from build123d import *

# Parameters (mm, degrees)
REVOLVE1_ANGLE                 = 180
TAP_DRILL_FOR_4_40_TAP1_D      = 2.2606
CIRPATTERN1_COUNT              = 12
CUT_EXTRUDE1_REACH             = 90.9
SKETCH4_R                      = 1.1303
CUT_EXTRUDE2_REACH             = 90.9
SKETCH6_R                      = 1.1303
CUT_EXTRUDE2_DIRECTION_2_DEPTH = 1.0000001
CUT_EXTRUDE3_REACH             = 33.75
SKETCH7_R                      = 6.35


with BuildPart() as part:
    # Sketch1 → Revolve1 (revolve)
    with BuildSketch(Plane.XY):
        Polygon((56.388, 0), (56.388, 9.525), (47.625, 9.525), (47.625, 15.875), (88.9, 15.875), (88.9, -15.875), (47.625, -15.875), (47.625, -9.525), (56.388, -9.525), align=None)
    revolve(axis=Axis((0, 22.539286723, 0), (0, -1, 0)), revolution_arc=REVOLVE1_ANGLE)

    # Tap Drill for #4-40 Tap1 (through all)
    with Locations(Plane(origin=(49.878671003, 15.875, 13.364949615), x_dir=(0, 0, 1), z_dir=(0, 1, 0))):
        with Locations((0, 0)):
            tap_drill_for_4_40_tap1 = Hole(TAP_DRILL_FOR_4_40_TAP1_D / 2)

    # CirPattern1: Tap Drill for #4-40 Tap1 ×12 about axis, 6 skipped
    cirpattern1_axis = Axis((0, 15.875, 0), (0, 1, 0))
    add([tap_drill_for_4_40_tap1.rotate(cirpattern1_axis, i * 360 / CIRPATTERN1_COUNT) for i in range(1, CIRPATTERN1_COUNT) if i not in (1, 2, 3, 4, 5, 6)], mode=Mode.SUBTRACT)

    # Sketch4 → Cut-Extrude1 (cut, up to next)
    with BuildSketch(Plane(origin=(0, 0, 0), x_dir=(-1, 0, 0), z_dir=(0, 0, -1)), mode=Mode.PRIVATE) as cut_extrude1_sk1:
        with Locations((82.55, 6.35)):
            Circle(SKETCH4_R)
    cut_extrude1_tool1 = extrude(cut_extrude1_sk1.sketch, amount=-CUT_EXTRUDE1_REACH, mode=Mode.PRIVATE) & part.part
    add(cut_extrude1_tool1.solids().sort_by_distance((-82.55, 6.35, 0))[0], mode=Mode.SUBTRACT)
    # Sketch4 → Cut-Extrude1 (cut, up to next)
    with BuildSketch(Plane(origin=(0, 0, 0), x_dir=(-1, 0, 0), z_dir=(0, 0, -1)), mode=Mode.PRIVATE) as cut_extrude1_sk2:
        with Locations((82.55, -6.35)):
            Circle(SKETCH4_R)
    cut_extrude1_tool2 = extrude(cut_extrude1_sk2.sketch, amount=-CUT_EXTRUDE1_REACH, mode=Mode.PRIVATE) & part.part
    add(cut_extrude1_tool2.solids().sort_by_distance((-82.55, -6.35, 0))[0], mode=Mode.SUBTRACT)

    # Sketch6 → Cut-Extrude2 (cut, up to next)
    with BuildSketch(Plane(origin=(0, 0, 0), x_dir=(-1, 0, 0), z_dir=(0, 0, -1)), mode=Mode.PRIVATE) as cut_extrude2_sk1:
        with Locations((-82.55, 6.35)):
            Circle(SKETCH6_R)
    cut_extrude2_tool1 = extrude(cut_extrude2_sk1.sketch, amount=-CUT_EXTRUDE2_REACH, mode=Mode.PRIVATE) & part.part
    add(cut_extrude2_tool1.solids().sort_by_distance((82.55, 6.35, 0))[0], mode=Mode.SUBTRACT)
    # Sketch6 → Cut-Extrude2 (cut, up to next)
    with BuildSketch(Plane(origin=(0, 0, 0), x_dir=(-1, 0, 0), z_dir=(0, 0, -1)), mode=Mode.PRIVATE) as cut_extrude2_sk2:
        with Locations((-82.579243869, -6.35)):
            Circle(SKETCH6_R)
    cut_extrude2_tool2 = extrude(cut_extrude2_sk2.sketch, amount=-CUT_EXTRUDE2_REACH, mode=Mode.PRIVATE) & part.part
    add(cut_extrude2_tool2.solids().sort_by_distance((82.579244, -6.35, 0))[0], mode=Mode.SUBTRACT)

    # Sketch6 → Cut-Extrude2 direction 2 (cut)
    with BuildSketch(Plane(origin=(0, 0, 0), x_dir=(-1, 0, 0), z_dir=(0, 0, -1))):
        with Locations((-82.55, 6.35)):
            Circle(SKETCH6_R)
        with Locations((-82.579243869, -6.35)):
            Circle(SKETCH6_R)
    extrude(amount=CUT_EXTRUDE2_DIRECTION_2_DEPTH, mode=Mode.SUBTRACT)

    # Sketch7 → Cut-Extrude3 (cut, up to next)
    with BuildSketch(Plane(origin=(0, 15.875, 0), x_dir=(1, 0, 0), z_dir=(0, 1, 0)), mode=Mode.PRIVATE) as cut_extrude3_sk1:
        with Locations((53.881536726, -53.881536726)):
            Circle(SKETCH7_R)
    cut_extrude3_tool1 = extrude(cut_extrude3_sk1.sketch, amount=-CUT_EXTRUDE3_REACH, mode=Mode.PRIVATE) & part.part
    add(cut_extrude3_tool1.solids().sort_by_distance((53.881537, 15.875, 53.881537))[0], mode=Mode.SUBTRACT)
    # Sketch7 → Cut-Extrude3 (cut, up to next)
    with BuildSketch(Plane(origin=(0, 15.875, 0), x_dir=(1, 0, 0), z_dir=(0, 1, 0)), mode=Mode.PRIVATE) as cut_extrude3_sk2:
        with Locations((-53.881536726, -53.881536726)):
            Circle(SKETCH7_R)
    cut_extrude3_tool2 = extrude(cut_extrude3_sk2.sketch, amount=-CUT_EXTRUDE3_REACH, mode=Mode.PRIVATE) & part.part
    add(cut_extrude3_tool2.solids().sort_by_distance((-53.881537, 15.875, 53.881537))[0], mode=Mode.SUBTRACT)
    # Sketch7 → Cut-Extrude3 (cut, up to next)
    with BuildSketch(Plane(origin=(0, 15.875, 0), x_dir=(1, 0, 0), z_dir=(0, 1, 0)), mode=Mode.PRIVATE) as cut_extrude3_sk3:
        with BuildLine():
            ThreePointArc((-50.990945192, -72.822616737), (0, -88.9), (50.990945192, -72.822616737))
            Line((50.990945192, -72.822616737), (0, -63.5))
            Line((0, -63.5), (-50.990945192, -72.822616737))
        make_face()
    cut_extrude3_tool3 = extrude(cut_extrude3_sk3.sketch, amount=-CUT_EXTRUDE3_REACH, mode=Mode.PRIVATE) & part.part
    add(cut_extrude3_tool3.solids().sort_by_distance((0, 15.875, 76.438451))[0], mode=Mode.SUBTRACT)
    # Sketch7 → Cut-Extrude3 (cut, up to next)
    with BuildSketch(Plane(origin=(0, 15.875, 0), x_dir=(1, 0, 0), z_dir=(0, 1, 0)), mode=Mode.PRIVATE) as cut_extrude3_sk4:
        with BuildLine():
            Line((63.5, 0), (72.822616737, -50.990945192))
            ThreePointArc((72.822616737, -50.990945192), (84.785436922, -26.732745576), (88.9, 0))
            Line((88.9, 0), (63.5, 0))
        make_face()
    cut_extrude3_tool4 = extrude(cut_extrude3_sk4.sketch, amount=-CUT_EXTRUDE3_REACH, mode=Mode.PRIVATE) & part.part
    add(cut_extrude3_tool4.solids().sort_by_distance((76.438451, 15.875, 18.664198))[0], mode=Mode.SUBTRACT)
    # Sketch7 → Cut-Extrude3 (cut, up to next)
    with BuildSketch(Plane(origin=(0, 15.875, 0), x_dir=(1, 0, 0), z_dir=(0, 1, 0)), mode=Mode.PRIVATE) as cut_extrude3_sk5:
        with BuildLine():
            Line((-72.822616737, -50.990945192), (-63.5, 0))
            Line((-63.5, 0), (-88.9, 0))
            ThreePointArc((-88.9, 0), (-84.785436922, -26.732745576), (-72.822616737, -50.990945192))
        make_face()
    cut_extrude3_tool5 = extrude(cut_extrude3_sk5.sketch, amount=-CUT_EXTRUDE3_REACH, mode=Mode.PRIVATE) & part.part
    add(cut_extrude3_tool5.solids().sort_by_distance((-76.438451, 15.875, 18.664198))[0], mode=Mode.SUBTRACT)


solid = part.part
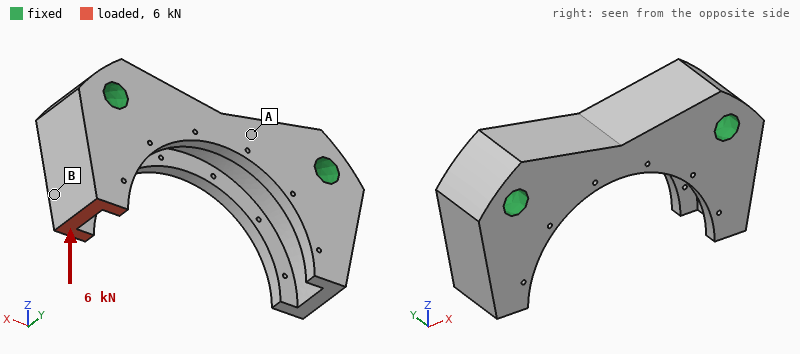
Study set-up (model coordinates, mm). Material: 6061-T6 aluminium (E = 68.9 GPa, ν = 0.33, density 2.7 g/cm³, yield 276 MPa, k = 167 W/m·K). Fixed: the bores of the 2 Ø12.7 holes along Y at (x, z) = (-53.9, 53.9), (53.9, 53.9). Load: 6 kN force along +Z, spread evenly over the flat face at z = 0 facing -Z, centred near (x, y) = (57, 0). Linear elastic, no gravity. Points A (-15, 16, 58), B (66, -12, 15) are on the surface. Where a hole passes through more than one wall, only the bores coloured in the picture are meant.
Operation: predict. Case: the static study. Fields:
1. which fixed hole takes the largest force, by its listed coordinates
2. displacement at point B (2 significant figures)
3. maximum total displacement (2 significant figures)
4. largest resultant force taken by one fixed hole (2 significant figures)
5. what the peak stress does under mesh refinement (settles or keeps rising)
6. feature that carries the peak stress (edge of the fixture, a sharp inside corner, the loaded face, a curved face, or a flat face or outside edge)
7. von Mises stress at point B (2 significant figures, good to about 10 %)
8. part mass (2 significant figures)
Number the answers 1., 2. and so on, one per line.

1. (53.9, 53.9)
2. 6.5 µm
3. 9.7 µm
4. 6.0 kN
5. keeps rising
6. a sharp inside corner
7. 10 MPa
8. 390 g
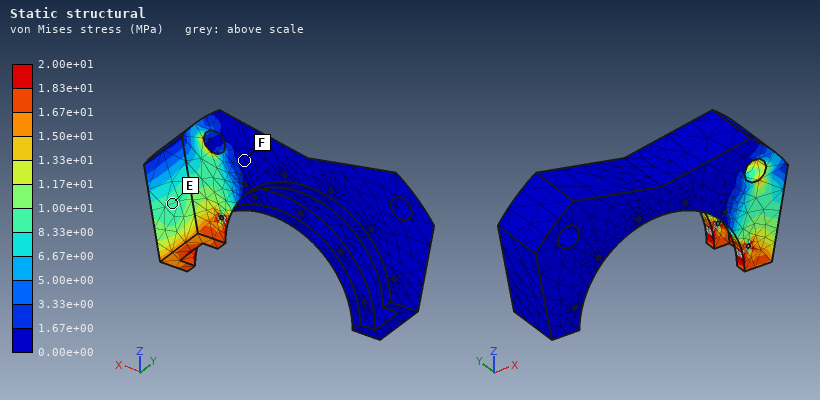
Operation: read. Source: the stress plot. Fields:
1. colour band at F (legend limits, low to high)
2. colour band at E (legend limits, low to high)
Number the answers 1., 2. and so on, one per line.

1. 0.00e+00 to 1.67e+00 MPa
2. 8.33e+00 to 1.00e+01 MPa
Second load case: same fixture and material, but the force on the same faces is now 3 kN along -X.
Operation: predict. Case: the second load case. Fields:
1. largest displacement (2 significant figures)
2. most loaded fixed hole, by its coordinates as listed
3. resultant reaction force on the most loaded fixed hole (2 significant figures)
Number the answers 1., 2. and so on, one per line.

1. 60 µm
2. (53.9, 53.9)
3. 3.1 kN
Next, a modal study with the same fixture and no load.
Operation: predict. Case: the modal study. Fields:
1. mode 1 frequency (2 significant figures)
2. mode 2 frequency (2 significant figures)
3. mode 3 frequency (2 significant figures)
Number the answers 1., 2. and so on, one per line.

1. 7900 Hz
2. 9700 Hz
3. 10000 Hz
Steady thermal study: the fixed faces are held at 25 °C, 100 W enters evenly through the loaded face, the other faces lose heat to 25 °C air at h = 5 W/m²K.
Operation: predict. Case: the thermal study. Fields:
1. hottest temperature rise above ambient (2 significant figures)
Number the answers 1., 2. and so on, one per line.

1. 52 K
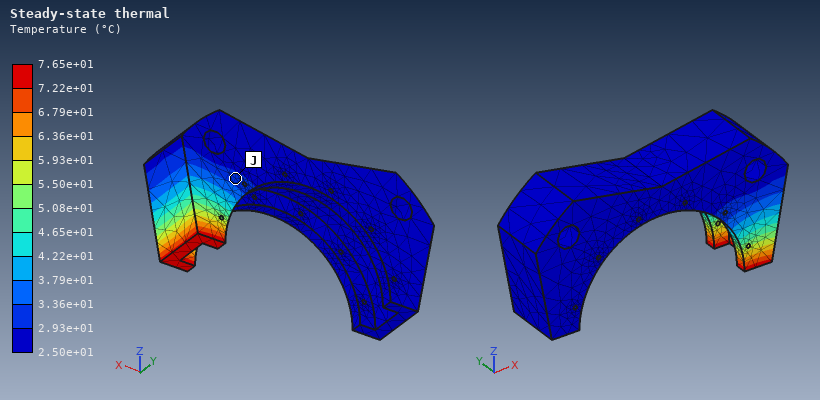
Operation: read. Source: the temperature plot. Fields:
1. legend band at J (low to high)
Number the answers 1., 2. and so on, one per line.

1. 2.93e+01 to 3.36e+01 °C
